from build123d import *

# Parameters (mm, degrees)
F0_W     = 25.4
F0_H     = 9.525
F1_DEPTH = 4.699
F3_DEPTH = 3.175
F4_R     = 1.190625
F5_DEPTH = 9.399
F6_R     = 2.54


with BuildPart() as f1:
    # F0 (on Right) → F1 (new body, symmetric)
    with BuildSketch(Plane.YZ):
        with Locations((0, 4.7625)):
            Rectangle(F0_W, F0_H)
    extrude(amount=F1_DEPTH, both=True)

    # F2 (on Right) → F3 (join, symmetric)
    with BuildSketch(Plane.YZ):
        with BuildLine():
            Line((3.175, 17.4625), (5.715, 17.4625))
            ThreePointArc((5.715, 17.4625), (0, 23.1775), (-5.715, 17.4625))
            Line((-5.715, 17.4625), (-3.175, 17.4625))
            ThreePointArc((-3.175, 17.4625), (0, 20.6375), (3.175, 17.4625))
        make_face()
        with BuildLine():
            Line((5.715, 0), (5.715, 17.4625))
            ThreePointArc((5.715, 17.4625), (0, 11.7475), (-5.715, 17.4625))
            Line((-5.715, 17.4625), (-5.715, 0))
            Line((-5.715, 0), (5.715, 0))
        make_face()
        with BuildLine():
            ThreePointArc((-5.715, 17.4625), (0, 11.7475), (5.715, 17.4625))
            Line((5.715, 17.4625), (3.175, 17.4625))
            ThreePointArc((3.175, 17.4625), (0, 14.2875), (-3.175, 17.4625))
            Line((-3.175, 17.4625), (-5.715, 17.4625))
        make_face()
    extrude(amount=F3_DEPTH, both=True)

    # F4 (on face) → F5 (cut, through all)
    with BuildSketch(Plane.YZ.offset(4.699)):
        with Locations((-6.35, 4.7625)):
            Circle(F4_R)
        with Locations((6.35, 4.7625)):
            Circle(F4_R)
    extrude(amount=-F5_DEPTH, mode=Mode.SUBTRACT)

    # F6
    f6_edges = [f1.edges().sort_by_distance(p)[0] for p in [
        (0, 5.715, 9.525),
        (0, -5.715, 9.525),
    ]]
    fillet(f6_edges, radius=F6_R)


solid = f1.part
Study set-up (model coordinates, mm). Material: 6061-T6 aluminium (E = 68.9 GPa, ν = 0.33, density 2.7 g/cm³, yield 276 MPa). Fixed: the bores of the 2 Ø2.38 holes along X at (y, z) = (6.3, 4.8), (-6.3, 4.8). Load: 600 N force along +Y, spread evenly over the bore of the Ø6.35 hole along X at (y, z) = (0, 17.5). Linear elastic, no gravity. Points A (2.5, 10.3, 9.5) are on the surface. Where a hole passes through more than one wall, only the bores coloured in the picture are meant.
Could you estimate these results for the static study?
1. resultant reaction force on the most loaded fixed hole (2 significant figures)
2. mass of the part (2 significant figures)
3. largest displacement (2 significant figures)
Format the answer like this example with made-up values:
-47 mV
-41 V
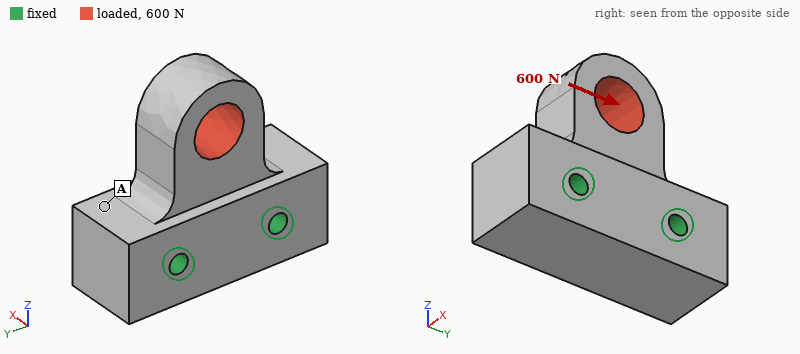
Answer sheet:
630 N
7.9 g
16 µm
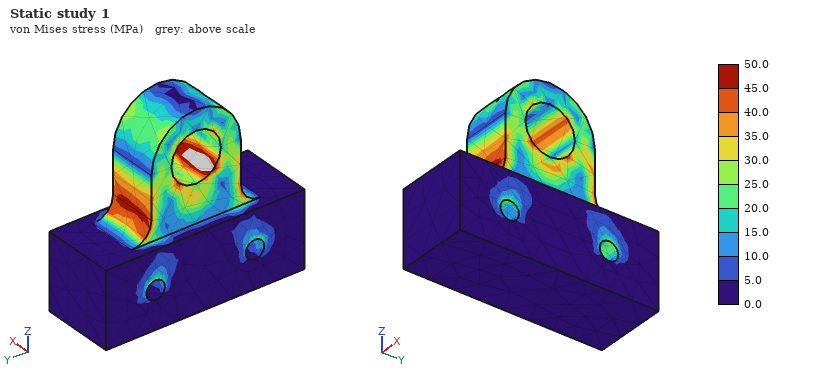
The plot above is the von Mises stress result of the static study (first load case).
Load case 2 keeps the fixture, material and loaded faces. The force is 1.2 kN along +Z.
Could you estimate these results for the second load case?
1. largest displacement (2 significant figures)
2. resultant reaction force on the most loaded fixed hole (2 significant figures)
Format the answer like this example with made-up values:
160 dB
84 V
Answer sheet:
6.8 µm
620 N
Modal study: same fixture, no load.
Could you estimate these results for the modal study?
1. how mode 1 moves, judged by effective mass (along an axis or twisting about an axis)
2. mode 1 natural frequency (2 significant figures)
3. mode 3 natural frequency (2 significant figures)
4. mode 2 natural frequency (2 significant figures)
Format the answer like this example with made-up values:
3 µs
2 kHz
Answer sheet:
along X
22 kHz
46 kHz
31 kHz
